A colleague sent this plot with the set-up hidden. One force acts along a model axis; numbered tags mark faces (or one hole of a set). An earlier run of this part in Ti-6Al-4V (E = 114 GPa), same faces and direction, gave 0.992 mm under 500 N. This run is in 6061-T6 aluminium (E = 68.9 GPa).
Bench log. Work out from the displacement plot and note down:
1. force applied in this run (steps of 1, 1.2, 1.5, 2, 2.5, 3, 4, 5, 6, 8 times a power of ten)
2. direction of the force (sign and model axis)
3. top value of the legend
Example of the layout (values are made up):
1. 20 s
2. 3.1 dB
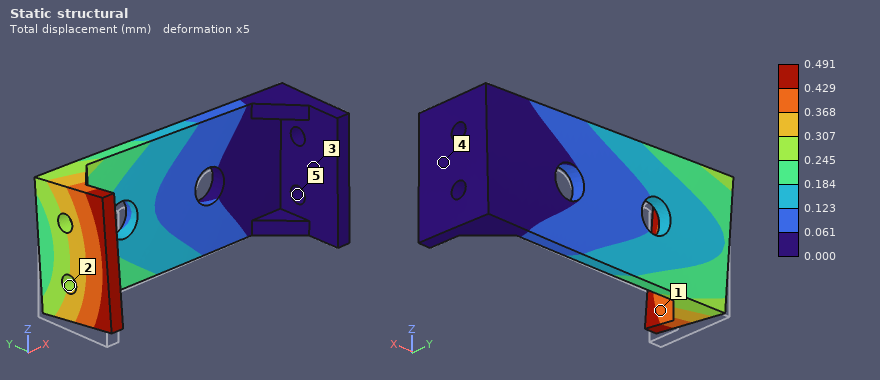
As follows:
1. 150 N
2. +Z
3. 0.491 mm
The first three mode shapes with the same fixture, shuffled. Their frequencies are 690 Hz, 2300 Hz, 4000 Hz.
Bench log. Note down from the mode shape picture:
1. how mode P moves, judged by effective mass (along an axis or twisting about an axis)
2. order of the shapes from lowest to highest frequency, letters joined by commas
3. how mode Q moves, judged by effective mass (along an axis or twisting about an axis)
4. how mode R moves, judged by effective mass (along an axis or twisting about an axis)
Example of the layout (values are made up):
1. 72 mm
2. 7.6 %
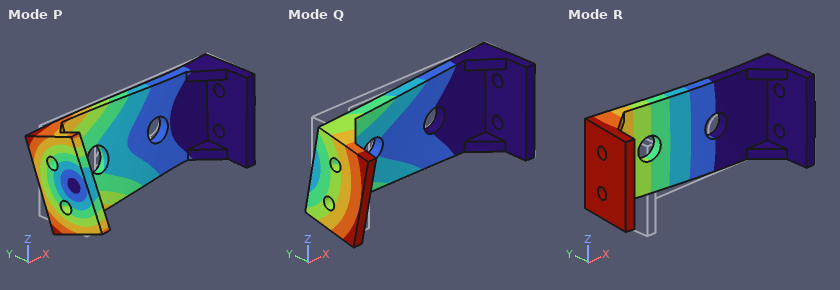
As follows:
1. along Z
2. R, Q, P
3. along Z
4. along Y
